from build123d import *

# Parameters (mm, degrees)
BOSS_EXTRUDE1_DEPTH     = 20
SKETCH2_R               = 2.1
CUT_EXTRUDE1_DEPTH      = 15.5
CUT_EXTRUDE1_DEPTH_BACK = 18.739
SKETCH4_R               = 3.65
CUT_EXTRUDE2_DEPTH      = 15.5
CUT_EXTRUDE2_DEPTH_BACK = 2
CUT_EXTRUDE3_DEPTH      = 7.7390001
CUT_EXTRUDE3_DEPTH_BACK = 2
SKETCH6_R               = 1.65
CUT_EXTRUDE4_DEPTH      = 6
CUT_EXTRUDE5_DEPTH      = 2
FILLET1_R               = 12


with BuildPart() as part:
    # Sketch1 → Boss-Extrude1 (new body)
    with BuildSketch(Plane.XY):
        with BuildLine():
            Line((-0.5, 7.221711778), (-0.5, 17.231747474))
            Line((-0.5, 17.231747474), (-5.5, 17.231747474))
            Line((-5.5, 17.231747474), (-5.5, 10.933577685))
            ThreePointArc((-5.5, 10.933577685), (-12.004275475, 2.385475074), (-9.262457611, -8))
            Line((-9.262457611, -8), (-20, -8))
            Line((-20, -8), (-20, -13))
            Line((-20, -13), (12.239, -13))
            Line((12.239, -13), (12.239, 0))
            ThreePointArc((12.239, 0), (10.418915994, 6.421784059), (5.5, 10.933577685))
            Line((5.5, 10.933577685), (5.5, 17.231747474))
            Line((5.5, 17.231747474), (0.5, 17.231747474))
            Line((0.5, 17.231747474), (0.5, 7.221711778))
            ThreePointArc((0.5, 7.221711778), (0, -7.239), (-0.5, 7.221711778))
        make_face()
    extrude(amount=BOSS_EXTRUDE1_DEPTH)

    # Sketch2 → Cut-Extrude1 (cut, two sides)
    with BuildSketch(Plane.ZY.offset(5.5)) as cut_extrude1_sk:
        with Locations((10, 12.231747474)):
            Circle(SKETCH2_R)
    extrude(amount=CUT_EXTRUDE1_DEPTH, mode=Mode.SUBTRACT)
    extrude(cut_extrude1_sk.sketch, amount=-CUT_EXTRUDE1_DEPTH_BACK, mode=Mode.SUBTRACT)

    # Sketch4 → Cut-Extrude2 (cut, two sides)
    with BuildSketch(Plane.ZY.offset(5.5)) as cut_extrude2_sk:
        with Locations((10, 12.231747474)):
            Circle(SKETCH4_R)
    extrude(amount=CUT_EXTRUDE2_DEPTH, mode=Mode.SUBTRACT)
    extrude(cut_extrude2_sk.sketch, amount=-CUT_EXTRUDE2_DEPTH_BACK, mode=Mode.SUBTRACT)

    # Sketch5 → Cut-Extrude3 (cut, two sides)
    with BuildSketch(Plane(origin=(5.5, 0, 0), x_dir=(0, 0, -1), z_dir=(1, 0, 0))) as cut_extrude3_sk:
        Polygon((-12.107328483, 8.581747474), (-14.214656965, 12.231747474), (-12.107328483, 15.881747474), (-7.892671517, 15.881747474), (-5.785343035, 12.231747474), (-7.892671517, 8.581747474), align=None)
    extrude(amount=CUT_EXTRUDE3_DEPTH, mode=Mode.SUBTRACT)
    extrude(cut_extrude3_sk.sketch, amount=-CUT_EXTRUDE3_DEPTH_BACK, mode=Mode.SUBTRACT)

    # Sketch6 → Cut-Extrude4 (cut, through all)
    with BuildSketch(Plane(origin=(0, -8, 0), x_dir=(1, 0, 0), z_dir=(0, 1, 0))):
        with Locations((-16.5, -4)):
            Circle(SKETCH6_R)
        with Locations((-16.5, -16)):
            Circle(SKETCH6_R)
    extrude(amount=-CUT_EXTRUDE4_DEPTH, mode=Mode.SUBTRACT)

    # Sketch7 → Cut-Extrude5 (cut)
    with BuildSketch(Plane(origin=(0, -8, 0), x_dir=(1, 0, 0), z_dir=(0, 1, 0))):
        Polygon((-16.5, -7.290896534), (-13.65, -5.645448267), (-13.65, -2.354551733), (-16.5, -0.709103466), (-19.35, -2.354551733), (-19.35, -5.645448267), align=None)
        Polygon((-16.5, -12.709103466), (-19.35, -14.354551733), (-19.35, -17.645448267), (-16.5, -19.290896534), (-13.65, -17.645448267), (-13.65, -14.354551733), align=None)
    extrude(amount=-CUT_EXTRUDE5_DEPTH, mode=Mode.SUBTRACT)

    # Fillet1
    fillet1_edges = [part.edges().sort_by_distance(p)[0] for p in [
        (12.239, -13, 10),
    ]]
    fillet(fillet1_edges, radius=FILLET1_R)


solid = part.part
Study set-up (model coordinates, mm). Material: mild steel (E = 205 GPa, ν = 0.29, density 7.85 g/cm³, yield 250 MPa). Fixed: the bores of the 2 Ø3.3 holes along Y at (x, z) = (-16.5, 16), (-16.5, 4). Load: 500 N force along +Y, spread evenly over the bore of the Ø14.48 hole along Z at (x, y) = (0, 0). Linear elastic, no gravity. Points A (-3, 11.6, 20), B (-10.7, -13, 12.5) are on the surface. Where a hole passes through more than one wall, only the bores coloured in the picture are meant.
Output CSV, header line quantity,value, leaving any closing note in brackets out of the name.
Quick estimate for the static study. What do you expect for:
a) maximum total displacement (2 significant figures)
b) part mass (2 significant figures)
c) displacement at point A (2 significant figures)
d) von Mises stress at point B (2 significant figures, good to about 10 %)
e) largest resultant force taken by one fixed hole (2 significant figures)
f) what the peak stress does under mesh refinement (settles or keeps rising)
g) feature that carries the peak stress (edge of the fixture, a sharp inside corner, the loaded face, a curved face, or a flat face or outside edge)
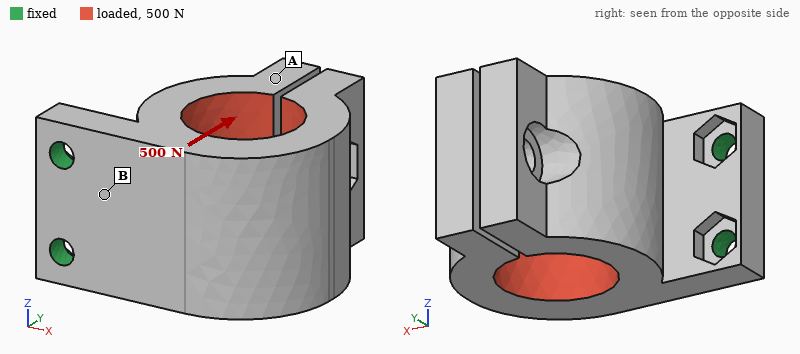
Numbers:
quantity,value
maximum total displacement,74 µm
part mass,65 g
displacement at point A,56 µm
von Mises stress at point B,60 MPa
largest resultant force taken by one fixed hole,250 N
what the peak stress does under mesh refinement,keeps rising
feature that carries the peak stress,edge of the fixture
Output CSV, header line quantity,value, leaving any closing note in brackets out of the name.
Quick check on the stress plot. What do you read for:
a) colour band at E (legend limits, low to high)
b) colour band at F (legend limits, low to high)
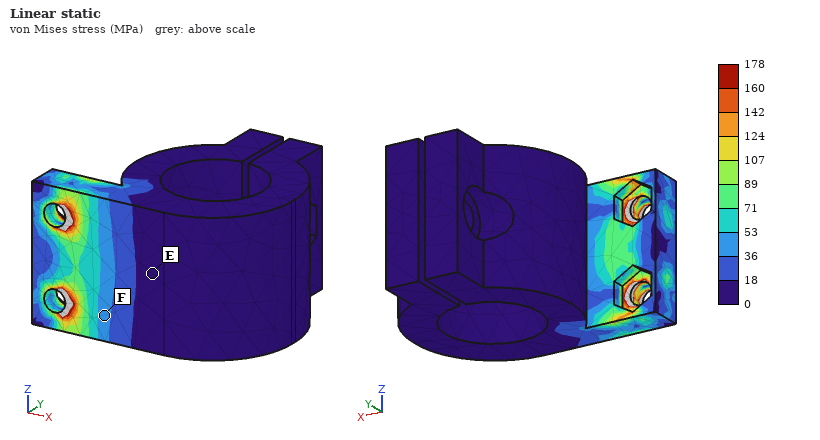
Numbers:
quantity,value
colour band at E,0 to 18 MPa
colour band at F,36 to 53 MPa
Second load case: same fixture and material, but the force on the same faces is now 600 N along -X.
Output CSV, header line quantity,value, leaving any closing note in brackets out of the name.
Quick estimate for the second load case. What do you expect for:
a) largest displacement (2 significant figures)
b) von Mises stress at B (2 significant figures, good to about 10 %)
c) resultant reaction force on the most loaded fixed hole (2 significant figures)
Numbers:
quantity,value
largest displacement,88 µm
von Mises stress at B,64 MPa
resultant reaction force on the most loaded fixed hole,300 N
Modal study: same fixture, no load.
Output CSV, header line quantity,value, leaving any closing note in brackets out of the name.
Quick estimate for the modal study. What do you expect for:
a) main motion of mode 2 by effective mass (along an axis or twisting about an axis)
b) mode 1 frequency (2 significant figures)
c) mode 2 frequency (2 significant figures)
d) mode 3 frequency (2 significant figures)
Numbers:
quantity,value
main motion of mode 2 by effective mass,along Z
mode 1 frequency,1700 Hz
mode 2 frequency,3700 Hz
mode 3 frequency,4700 Hz
